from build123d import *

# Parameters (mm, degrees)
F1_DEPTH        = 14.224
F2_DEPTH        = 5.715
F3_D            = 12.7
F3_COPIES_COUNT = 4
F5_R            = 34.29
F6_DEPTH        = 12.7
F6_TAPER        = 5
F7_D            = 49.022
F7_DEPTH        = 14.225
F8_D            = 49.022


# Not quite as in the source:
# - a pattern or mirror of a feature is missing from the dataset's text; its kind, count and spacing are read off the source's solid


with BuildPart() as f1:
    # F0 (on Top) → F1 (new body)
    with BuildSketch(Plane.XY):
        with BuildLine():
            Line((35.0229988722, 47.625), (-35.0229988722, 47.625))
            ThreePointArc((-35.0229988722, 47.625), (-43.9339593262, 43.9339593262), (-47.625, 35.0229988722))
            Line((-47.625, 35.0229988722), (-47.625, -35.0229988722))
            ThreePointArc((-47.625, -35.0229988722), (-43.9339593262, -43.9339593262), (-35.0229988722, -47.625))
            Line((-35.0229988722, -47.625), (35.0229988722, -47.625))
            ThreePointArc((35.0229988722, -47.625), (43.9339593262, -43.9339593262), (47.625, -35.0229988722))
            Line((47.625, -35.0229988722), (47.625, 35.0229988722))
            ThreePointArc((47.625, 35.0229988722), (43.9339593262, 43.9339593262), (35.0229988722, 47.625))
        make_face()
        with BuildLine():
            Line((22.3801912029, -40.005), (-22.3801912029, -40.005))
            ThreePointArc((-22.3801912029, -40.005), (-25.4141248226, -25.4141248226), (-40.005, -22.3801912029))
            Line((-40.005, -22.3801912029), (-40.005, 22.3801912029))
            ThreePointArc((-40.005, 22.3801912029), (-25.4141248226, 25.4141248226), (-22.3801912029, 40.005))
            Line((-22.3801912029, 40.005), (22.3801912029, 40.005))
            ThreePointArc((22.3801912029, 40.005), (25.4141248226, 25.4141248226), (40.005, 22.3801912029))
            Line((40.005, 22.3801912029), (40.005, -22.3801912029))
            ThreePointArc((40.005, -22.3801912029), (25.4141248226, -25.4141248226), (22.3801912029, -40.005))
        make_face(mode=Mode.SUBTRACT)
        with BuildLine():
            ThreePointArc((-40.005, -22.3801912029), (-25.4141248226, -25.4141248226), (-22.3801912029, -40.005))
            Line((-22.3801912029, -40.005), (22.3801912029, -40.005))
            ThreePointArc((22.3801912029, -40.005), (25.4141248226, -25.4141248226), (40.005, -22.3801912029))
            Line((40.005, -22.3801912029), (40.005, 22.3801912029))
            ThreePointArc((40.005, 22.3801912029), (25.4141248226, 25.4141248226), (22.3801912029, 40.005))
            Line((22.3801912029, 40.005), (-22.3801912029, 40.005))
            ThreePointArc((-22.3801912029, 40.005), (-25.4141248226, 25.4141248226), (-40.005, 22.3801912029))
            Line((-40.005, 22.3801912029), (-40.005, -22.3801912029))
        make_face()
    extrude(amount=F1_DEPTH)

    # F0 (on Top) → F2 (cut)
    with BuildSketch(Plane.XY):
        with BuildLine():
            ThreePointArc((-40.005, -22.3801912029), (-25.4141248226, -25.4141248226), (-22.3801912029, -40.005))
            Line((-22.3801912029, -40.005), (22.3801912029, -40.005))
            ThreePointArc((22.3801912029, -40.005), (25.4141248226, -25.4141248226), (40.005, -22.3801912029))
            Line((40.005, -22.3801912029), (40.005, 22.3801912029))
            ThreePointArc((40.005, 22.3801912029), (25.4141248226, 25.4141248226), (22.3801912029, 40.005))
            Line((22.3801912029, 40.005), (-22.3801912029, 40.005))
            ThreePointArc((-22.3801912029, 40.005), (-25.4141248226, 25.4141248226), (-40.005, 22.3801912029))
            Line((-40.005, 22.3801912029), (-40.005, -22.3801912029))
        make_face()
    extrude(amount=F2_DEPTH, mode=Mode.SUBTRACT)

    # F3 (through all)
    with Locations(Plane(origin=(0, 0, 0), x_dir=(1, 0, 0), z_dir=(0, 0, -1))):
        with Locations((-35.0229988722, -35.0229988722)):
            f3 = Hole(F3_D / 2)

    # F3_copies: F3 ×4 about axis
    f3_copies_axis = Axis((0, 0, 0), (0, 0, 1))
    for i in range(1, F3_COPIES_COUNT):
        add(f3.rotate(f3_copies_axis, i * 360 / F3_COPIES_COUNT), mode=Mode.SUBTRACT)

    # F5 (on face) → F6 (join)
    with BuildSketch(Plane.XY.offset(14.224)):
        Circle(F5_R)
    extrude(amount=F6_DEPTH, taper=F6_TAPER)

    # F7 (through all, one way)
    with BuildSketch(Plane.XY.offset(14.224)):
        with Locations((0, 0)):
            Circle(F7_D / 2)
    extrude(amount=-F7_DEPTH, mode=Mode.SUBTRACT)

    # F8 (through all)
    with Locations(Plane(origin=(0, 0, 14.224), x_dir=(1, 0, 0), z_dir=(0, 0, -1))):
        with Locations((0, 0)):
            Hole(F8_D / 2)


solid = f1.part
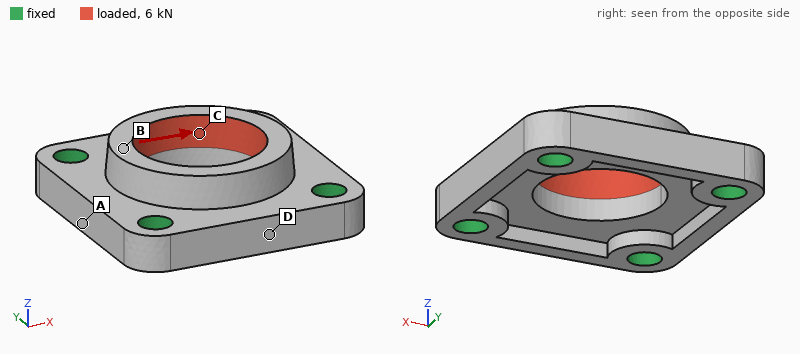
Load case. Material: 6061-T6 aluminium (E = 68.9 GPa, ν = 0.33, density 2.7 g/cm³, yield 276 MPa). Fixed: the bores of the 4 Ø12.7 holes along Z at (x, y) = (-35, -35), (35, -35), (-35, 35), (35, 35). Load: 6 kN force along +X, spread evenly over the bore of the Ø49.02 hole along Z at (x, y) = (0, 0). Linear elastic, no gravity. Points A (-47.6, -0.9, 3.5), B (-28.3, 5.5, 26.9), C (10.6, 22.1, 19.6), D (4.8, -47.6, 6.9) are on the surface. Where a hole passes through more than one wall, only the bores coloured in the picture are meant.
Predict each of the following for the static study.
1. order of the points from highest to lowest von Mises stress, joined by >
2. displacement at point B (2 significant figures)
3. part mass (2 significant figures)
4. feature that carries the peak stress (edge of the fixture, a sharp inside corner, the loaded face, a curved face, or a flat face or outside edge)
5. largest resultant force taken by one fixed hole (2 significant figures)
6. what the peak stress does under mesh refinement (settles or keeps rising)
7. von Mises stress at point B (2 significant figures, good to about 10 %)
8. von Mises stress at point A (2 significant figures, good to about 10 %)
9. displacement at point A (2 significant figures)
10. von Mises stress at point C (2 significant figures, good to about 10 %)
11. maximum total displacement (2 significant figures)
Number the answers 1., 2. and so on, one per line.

1. C > B > A > D
2. 8.0 µm
3. 260 g
4. edge of the fixture
5. 1.6 kN
6. keeps rising
7. 8.2 MPa
8. 4.6 MPa
9. 3.1 µm
10. 11 MPa
11. 8.8 µm
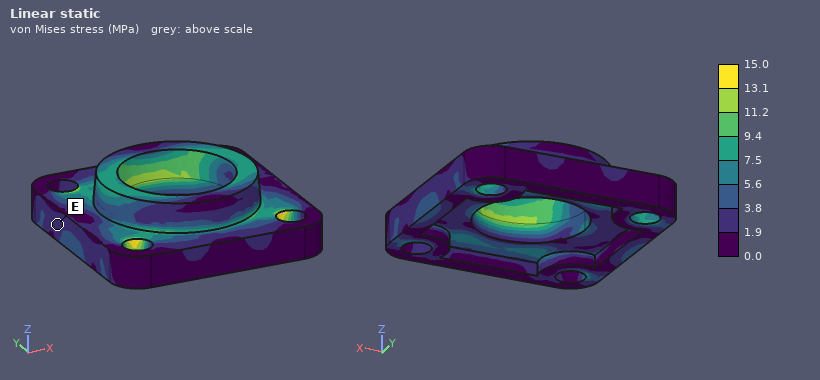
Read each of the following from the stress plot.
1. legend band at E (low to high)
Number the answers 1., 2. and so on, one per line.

1. 1.9 to 3.8 MPa
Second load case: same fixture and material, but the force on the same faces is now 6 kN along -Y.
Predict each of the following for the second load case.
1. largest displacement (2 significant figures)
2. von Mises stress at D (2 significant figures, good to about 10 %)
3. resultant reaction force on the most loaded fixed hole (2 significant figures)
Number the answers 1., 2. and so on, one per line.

1. 8.7 µm
2. 3.9 MPa
3. 1.6 kN
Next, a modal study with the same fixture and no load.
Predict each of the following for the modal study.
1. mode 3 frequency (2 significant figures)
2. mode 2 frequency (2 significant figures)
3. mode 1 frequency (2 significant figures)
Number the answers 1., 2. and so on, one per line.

1. 15 kHz
2. 14 kHz
3. 13 kHz
